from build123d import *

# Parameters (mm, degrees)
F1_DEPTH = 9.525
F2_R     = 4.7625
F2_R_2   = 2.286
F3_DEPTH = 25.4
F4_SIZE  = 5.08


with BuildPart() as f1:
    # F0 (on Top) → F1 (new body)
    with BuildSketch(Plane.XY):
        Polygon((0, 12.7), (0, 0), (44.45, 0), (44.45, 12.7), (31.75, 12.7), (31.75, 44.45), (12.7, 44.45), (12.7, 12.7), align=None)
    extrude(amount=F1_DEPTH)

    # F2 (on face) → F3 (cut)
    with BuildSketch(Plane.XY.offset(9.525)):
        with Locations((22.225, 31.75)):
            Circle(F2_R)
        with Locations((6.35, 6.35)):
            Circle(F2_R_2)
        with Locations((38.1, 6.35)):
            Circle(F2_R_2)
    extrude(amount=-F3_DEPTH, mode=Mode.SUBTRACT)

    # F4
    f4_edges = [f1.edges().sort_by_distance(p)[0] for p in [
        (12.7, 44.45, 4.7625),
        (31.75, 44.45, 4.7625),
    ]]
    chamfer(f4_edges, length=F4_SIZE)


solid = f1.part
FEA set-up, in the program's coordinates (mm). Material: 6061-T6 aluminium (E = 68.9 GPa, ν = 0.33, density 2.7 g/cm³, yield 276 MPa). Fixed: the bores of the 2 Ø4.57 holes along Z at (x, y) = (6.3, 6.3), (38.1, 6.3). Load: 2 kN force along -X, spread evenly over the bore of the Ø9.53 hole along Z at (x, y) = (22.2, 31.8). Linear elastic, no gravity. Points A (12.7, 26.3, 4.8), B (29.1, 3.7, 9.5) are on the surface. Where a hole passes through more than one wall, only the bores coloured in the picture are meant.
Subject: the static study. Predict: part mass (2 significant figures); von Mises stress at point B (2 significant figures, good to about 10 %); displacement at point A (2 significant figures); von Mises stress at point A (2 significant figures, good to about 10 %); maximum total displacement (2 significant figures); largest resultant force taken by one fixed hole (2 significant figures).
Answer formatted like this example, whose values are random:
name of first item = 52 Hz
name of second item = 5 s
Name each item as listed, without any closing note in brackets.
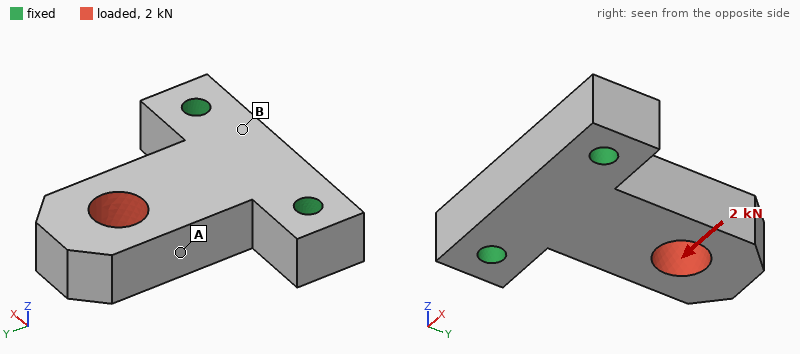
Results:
part mass = 27 g
von Mises stress at point B = 10 MPa
displacement at point A = 31 µm
von Mises stress at point A = 39 MPa
maximum total displacement = 68 µm
largest resultant force taken by one fixed hole = 2.0 kN
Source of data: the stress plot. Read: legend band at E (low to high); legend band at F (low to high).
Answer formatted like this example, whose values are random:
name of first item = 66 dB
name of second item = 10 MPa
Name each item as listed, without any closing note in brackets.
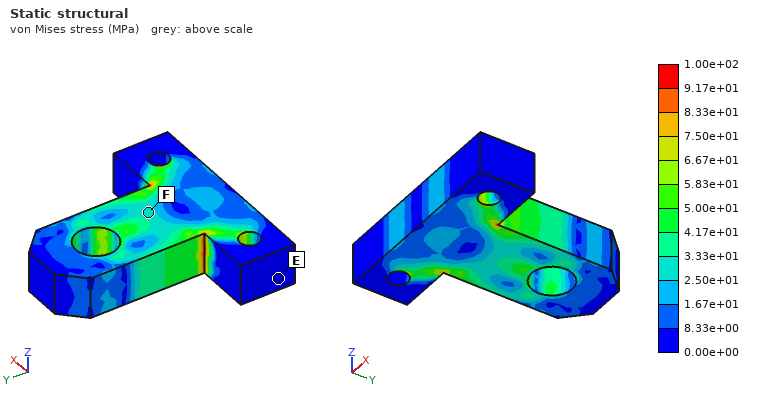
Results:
legend band at E = 0.00e+00 to 8.33e+00 MPa
legend band at F = 2.50e+01 to 3.33e+01 MPa
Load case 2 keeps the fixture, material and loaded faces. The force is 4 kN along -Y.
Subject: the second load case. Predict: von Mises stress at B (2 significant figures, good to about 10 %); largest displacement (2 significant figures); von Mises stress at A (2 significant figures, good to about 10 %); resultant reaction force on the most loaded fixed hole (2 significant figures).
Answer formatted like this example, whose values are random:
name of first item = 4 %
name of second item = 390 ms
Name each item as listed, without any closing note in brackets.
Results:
von Mises stress at B = 17 MPa
largest displacement = 20 µm
von Mises stress at A = 23 MPa
resultant reaction force on the most loaded fixed hole = 2.1 kN
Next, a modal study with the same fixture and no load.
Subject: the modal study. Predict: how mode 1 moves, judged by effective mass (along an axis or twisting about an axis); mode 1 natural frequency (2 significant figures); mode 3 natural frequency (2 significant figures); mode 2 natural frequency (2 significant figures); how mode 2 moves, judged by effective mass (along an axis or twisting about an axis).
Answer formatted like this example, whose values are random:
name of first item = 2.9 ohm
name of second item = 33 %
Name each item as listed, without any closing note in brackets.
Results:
how mode 1 moves, judged by effective mass = along Z
mode 1 natural frequency = 4700 Hz
mode 3 natural frequency = 17 kHz
mode 2 natural frequency = 10 kHz
how mode 2 moves, judged by effective mass = along X
